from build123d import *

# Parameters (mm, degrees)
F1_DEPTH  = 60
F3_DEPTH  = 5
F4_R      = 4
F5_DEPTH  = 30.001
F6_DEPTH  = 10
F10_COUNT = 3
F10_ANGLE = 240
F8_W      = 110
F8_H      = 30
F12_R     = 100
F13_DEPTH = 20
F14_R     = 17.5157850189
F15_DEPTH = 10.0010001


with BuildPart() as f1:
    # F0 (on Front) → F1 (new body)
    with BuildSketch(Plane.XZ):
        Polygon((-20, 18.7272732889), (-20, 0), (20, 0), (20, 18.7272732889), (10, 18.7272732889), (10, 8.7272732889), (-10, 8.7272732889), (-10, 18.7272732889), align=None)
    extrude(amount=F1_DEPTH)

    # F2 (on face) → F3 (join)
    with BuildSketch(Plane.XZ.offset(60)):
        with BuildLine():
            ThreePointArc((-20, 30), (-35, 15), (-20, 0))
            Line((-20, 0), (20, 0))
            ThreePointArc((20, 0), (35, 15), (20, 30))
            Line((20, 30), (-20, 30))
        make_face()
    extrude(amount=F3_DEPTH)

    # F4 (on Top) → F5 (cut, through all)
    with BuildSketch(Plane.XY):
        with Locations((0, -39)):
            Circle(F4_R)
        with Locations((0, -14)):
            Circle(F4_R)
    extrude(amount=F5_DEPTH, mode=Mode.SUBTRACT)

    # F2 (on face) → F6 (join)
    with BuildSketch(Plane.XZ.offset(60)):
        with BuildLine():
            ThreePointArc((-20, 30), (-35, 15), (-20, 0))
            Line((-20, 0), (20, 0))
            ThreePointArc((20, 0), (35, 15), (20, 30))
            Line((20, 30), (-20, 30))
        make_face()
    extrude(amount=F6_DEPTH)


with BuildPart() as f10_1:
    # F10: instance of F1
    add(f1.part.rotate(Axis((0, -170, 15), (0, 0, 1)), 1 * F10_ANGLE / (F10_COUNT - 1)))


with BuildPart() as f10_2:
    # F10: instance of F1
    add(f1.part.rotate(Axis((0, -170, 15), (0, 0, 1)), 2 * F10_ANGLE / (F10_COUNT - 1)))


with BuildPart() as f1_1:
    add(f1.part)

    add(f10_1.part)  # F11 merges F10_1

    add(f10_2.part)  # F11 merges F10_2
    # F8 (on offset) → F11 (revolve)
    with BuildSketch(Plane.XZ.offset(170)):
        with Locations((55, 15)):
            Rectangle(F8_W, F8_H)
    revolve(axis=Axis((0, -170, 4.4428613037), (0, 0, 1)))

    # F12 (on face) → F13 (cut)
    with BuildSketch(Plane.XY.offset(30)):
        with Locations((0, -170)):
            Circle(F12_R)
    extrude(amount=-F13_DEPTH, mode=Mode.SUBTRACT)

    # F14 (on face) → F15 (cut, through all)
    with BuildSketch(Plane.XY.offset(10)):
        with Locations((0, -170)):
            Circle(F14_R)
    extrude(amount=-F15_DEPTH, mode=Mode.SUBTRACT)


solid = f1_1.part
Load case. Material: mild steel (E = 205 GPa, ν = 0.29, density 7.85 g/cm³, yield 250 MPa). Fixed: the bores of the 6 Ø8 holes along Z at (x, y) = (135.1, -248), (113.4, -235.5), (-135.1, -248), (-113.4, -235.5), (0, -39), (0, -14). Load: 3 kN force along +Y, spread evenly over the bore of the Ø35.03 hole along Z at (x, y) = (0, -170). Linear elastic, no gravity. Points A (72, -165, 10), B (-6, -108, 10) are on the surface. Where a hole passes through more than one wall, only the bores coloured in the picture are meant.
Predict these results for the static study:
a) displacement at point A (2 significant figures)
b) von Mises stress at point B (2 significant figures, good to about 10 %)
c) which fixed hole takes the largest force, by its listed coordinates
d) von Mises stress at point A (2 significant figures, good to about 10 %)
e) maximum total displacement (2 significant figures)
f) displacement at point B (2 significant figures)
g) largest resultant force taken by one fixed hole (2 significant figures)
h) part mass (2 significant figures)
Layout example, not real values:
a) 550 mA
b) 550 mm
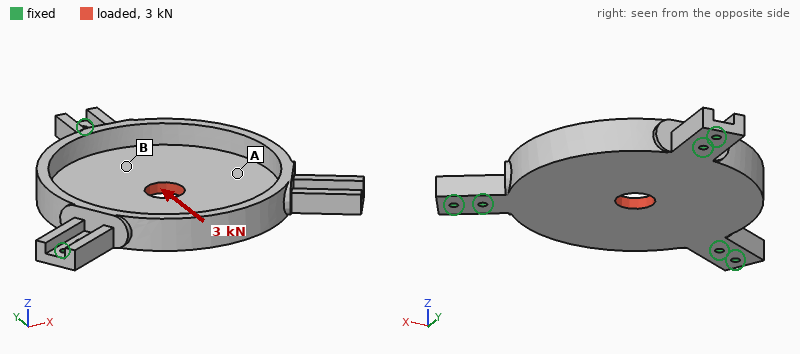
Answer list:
a) 1.2 µm
b) 2.8 MPa
c) (0, -39)
d) 0.94 MPa
e) 2.1 µm
f) 1.0 µm
g) 1.1 kN
h) 4.8 kg
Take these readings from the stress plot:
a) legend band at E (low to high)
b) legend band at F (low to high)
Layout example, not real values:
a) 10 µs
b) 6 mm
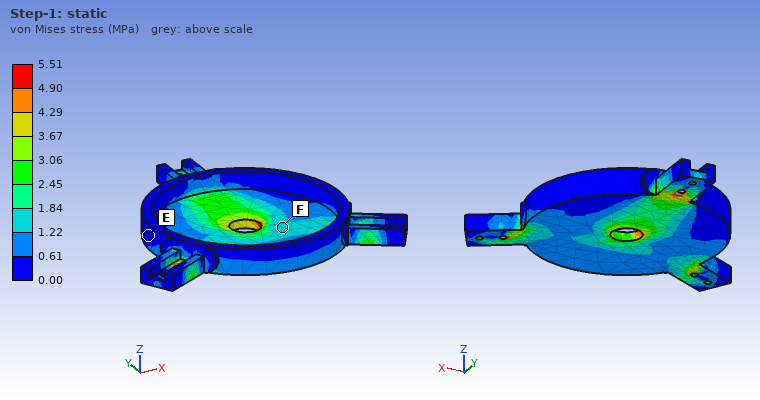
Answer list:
a) 0.00 to 0.61 MPa
b) 1.22 to 1.84 MPa
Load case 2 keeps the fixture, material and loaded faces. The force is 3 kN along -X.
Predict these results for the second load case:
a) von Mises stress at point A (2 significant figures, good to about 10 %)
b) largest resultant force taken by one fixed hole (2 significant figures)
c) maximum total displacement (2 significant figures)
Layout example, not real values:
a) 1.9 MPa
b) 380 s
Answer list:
a) 1.3 MPa
b) 1.0 kN
c) 2.0 µm
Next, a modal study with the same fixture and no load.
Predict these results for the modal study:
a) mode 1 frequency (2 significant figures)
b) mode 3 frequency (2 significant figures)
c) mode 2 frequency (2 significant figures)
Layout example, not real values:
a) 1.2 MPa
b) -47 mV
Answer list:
a) 1200 Hz
b) 1200 Hz
c) 1200 Hz
